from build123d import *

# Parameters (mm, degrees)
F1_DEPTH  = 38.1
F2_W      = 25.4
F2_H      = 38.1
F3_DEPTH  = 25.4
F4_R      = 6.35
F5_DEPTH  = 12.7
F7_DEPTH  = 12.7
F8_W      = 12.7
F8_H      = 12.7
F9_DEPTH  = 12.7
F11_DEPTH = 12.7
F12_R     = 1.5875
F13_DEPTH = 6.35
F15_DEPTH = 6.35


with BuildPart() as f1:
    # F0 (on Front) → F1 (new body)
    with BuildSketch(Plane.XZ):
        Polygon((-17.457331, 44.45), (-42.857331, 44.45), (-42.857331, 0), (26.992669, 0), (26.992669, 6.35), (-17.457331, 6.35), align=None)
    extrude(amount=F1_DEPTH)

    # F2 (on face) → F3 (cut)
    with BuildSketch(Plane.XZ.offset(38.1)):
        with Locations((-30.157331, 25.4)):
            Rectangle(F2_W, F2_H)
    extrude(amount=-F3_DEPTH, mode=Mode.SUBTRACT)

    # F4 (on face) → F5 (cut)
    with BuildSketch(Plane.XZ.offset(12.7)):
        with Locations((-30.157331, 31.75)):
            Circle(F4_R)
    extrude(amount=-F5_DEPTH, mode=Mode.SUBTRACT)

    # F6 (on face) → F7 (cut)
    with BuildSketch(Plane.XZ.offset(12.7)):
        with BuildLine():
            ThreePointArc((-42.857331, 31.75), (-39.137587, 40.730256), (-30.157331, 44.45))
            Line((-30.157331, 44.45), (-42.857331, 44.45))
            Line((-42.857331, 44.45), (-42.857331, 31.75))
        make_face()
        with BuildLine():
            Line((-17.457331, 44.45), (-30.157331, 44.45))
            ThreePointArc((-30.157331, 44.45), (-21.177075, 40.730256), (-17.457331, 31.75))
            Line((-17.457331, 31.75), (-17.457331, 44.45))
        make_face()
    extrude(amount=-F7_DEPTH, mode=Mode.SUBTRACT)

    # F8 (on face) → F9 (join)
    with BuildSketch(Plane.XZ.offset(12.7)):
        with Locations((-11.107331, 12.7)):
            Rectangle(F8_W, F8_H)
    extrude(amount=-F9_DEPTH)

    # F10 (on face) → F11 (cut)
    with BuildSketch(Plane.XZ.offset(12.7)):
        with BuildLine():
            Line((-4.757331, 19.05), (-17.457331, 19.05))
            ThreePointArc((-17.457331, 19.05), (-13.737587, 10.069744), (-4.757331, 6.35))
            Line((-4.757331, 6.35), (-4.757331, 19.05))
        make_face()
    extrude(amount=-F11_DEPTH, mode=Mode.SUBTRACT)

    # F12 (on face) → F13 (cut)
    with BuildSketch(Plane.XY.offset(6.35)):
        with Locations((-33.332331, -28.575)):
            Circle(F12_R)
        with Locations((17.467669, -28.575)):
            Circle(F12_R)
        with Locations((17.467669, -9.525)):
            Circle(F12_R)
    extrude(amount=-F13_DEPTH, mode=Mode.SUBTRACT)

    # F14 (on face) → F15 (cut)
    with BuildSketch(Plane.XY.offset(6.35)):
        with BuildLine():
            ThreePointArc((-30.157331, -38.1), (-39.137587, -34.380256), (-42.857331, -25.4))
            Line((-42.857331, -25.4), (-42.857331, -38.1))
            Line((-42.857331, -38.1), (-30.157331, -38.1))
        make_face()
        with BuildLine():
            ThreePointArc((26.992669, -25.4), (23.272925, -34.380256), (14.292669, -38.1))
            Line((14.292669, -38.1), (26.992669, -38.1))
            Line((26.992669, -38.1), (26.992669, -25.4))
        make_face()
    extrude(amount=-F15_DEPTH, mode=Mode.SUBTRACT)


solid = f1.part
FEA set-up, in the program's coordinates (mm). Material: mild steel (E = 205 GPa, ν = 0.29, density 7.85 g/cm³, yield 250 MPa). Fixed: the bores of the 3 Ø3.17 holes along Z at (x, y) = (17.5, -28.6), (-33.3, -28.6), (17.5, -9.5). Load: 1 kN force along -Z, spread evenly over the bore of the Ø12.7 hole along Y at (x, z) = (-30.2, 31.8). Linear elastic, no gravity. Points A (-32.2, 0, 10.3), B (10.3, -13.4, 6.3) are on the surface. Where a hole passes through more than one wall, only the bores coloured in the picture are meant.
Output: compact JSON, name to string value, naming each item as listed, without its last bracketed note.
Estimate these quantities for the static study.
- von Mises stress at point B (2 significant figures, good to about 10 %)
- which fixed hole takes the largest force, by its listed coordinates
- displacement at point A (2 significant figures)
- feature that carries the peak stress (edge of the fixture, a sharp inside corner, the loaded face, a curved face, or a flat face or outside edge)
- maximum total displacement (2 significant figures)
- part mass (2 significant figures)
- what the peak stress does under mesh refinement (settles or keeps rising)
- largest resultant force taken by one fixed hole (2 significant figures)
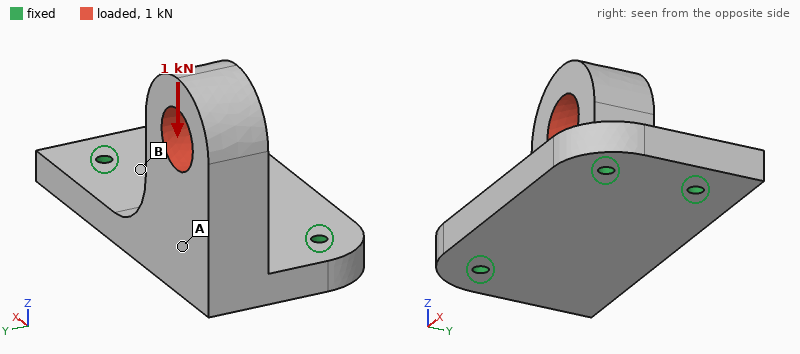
{"von Mises stress at point B": "26 MPa", "which fixed hole takes the largest force, by its listed coordinates": "(-33.3, -28.6)", "displacement at point A": "32 µm", "feature that carries the peak stress": "edge of the fixture", "maximum total displacement": "60 µm", "part mass": "210 g", "what the peak stress does under mesh refinement": "keeps rising", "largest resultant force taken by one fixed hole": "840 N"}
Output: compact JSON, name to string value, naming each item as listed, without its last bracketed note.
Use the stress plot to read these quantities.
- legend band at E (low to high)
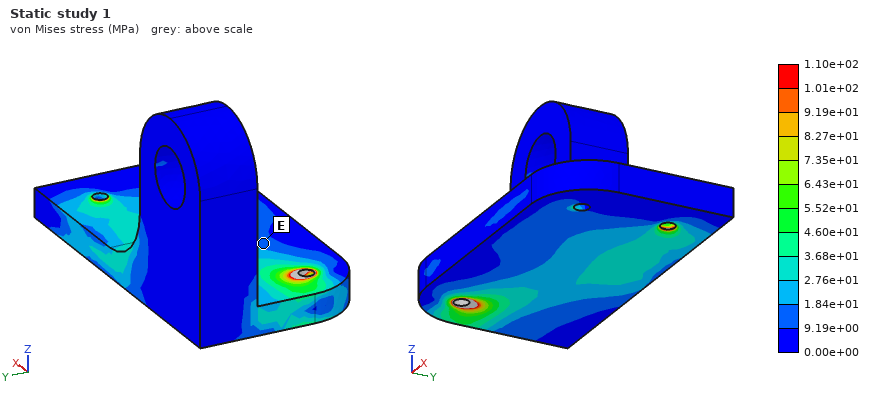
{"legend band at E": "9.19e+00 to 1.84e+01 MPa"}
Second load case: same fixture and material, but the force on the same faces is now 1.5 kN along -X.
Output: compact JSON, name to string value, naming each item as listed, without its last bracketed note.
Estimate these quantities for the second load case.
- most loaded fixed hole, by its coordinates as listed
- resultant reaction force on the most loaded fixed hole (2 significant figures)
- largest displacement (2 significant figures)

{"most loaded fixed hole, by its coordinates as listed": "(-33.3, -28.6)", "resultant reaction force on the most loaded fixed hole": "1.0 kN", "largest displacement": "69 µm"}
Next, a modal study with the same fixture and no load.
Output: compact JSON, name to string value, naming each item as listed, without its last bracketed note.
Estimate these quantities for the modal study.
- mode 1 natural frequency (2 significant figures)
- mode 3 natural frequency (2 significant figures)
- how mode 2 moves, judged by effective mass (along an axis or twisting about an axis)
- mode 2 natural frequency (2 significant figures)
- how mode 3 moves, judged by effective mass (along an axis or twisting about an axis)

{"mode 1 natural frequency": "2100 Hz", "mode 3 natural frequency": "6400 Hz", "how mode 2 moves, judged by effective mass": "along X", "mode 2 natural frequency": "4300 Hz", "how mode 3 moves, judged by effective mass": "along Z"}
